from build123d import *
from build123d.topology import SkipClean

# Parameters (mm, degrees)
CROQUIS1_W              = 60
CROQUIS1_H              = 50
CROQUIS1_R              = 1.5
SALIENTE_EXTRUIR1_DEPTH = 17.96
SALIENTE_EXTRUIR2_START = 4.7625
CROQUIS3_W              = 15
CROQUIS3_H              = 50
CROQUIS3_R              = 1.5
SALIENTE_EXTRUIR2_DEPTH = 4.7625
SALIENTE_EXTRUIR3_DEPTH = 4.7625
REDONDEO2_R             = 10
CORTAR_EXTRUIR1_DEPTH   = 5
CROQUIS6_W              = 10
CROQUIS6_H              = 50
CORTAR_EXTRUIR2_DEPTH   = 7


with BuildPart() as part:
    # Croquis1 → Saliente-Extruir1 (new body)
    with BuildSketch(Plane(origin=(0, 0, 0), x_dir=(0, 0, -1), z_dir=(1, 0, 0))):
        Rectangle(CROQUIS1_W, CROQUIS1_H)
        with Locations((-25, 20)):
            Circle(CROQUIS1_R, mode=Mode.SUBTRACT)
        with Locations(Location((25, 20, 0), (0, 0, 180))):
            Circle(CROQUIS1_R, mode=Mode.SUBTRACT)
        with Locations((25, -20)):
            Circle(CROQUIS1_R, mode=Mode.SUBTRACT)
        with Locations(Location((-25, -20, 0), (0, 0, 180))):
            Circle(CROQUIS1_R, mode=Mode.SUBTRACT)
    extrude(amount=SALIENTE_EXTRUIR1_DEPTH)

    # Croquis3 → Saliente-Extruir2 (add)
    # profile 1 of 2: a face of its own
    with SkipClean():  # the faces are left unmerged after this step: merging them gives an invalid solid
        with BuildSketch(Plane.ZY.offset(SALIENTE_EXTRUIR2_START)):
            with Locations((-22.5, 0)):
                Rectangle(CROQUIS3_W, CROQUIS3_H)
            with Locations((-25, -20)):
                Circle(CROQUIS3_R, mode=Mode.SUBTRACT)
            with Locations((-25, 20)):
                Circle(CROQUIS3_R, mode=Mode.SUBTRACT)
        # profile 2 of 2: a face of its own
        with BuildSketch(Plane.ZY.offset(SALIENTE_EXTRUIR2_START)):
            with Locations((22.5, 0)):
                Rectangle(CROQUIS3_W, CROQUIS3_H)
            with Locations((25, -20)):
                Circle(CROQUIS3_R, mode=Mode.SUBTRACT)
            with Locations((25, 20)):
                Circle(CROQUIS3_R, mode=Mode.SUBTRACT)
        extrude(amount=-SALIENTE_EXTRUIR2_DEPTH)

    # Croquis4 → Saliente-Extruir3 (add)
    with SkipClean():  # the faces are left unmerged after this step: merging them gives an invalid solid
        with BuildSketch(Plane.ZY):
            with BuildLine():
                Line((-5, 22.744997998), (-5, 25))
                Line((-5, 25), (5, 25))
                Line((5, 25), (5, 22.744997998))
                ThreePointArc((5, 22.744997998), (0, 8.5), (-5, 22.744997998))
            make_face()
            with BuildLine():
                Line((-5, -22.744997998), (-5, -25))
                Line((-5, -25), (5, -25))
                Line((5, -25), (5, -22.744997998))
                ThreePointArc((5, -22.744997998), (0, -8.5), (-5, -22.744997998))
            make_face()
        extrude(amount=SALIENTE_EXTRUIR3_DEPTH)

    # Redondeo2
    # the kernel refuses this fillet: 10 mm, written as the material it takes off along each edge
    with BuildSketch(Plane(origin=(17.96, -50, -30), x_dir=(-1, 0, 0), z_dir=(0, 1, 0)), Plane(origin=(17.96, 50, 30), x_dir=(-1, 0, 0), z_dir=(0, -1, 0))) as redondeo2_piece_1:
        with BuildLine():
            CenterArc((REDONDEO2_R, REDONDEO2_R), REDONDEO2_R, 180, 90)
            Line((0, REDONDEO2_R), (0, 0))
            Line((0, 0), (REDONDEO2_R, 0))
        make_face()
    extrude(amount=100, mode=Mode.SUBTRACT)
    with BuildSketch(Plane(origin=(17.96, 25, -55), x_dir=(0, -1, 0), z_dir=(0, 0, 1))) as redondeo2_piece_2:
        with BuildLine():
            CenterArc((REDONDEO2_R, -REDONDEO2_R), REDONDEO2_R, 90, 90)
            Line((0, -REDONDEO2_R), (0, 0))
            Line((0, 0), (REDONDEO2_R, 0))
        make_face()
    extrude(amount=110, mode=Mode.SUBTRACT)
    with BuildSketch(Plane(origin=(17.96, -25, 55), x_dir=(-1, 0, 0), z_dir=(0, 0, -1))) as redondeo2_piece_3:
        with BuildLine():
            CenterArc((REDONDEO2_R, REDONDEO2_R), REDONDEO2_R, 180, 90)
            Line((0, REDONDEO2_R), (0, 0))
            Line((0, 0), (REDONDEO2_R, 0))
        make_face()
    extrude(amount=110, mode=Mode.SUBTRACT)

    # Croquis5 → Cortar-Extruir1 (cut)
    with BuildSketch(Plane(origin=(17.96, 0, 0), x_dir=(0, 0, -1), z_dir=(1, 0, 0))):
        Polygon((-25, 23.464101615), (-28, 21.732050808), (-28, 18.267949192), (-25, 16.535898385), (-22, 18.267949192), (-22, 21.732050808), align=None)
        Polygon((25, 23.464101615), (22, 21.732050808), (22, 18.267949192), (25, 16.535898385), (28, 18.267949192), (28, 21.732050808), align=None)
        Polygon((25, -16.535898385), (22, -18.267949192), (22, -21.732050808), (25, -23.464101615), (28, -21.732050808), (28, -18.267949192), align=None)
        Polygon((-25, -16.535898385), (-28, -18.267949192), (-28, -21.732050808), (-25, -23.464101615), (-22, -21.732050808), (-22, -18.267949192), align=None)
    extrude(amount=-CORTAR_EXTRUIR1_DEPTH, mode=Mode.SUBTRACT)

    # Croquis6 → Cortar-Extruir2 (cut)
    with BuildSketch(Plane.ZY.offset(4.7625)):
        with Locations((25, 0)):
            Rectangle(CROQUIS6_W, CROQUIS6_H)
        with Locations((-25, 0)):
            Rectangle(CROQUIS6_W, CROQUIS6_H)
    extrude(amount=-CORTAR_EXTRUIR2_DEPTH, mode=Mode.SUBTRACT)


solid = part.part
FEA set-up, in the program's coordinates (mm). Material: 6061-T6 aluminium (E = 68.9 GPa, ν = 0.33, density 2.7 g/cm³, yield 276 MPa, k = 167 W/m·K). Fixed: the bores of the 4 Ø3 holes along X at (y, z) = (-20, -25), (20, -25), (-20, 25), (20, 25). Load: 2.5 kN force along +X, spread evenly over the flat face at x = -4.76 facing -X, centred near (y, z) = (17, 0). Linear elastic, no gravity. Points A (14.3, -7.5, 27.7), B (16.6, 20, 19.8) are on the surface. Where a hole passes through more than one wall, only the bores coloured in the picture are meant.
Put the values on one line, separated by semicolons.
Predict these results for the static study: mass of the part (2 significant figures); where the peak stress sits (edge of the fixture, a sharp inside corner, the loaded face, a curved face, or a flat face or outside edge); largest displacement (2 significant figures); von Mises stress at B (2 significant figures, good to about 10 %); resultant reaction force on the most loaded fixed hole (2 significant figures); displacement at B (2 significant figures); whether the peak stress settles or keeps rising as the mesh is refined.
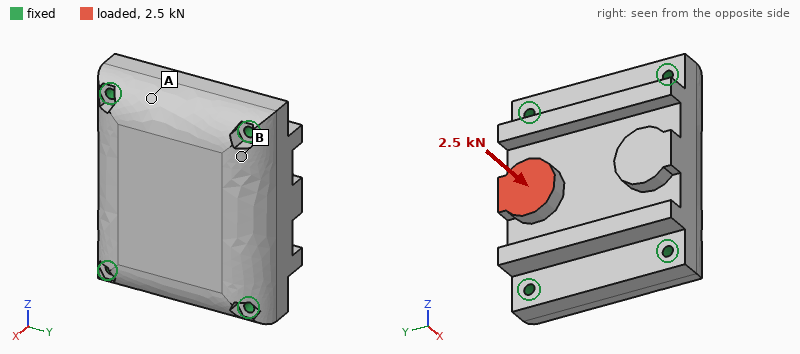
140 g; edge of the fixture; 12 µm; 8.9 MPa; 1.1 kN; 3.5 µm; keeps rising
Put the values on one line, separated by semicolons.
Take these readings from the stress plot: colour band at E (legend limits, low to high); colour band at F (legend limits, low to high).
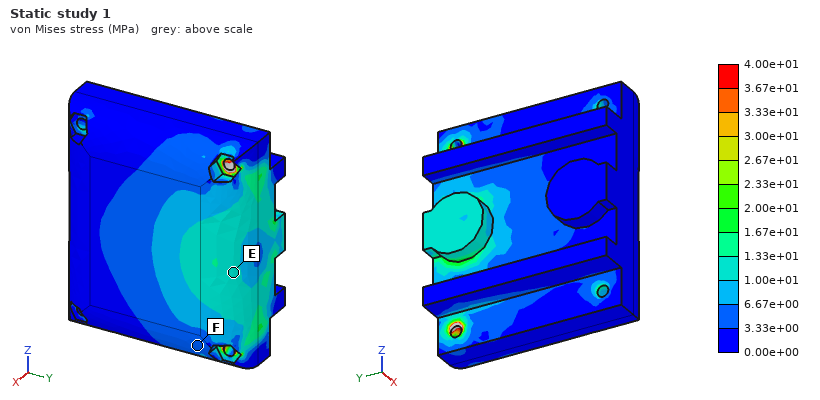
1.00e+01 to 1.33e+01 MPa; 3.33e+00 to 6.67e+00 MPa
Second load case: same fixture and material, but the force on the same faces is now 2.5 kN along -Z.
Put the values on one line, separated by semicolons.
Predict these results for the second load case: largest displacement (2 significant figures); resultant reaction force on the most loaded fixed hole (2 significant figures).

9.7 µm; 1.1 kN
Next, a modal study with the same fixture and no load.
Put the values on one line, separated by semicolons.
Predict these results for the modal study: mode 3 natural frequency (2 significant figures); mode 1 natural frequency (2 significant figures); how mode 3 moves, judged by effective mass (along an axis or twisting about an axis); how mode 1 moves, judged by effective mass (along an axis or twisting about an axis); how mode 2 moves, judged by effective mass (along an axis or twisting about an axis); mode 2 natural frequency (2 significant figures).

21 kHz; 14 kHz; along Y; along X; along Y; 18 kHz
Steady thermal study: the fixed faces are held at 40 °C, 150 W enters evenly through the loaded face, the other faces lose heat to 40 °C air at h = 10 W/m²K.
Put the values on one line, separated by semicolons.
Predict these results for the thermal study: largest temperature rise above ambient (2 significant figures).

63 K
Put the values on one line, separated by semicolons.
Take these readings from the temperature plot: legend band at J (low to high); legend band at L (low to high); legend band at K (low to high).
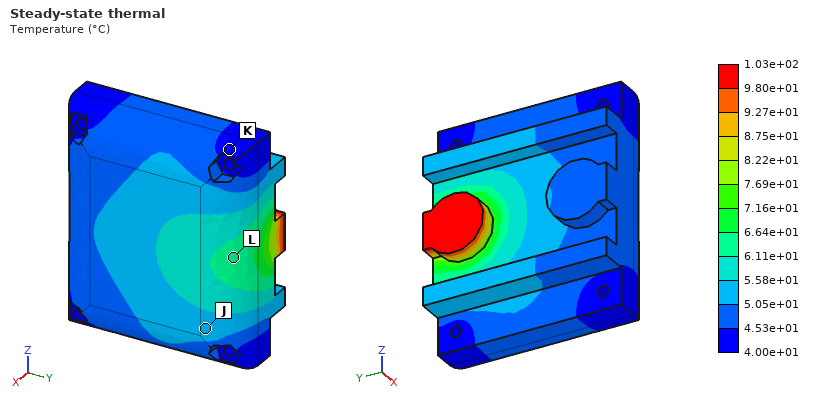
5.05e+01 to 5.58e+01 °C; 6.11e+01 to 6.64e+01 °C; 4.00e+01 to 4.53e+01 °C
